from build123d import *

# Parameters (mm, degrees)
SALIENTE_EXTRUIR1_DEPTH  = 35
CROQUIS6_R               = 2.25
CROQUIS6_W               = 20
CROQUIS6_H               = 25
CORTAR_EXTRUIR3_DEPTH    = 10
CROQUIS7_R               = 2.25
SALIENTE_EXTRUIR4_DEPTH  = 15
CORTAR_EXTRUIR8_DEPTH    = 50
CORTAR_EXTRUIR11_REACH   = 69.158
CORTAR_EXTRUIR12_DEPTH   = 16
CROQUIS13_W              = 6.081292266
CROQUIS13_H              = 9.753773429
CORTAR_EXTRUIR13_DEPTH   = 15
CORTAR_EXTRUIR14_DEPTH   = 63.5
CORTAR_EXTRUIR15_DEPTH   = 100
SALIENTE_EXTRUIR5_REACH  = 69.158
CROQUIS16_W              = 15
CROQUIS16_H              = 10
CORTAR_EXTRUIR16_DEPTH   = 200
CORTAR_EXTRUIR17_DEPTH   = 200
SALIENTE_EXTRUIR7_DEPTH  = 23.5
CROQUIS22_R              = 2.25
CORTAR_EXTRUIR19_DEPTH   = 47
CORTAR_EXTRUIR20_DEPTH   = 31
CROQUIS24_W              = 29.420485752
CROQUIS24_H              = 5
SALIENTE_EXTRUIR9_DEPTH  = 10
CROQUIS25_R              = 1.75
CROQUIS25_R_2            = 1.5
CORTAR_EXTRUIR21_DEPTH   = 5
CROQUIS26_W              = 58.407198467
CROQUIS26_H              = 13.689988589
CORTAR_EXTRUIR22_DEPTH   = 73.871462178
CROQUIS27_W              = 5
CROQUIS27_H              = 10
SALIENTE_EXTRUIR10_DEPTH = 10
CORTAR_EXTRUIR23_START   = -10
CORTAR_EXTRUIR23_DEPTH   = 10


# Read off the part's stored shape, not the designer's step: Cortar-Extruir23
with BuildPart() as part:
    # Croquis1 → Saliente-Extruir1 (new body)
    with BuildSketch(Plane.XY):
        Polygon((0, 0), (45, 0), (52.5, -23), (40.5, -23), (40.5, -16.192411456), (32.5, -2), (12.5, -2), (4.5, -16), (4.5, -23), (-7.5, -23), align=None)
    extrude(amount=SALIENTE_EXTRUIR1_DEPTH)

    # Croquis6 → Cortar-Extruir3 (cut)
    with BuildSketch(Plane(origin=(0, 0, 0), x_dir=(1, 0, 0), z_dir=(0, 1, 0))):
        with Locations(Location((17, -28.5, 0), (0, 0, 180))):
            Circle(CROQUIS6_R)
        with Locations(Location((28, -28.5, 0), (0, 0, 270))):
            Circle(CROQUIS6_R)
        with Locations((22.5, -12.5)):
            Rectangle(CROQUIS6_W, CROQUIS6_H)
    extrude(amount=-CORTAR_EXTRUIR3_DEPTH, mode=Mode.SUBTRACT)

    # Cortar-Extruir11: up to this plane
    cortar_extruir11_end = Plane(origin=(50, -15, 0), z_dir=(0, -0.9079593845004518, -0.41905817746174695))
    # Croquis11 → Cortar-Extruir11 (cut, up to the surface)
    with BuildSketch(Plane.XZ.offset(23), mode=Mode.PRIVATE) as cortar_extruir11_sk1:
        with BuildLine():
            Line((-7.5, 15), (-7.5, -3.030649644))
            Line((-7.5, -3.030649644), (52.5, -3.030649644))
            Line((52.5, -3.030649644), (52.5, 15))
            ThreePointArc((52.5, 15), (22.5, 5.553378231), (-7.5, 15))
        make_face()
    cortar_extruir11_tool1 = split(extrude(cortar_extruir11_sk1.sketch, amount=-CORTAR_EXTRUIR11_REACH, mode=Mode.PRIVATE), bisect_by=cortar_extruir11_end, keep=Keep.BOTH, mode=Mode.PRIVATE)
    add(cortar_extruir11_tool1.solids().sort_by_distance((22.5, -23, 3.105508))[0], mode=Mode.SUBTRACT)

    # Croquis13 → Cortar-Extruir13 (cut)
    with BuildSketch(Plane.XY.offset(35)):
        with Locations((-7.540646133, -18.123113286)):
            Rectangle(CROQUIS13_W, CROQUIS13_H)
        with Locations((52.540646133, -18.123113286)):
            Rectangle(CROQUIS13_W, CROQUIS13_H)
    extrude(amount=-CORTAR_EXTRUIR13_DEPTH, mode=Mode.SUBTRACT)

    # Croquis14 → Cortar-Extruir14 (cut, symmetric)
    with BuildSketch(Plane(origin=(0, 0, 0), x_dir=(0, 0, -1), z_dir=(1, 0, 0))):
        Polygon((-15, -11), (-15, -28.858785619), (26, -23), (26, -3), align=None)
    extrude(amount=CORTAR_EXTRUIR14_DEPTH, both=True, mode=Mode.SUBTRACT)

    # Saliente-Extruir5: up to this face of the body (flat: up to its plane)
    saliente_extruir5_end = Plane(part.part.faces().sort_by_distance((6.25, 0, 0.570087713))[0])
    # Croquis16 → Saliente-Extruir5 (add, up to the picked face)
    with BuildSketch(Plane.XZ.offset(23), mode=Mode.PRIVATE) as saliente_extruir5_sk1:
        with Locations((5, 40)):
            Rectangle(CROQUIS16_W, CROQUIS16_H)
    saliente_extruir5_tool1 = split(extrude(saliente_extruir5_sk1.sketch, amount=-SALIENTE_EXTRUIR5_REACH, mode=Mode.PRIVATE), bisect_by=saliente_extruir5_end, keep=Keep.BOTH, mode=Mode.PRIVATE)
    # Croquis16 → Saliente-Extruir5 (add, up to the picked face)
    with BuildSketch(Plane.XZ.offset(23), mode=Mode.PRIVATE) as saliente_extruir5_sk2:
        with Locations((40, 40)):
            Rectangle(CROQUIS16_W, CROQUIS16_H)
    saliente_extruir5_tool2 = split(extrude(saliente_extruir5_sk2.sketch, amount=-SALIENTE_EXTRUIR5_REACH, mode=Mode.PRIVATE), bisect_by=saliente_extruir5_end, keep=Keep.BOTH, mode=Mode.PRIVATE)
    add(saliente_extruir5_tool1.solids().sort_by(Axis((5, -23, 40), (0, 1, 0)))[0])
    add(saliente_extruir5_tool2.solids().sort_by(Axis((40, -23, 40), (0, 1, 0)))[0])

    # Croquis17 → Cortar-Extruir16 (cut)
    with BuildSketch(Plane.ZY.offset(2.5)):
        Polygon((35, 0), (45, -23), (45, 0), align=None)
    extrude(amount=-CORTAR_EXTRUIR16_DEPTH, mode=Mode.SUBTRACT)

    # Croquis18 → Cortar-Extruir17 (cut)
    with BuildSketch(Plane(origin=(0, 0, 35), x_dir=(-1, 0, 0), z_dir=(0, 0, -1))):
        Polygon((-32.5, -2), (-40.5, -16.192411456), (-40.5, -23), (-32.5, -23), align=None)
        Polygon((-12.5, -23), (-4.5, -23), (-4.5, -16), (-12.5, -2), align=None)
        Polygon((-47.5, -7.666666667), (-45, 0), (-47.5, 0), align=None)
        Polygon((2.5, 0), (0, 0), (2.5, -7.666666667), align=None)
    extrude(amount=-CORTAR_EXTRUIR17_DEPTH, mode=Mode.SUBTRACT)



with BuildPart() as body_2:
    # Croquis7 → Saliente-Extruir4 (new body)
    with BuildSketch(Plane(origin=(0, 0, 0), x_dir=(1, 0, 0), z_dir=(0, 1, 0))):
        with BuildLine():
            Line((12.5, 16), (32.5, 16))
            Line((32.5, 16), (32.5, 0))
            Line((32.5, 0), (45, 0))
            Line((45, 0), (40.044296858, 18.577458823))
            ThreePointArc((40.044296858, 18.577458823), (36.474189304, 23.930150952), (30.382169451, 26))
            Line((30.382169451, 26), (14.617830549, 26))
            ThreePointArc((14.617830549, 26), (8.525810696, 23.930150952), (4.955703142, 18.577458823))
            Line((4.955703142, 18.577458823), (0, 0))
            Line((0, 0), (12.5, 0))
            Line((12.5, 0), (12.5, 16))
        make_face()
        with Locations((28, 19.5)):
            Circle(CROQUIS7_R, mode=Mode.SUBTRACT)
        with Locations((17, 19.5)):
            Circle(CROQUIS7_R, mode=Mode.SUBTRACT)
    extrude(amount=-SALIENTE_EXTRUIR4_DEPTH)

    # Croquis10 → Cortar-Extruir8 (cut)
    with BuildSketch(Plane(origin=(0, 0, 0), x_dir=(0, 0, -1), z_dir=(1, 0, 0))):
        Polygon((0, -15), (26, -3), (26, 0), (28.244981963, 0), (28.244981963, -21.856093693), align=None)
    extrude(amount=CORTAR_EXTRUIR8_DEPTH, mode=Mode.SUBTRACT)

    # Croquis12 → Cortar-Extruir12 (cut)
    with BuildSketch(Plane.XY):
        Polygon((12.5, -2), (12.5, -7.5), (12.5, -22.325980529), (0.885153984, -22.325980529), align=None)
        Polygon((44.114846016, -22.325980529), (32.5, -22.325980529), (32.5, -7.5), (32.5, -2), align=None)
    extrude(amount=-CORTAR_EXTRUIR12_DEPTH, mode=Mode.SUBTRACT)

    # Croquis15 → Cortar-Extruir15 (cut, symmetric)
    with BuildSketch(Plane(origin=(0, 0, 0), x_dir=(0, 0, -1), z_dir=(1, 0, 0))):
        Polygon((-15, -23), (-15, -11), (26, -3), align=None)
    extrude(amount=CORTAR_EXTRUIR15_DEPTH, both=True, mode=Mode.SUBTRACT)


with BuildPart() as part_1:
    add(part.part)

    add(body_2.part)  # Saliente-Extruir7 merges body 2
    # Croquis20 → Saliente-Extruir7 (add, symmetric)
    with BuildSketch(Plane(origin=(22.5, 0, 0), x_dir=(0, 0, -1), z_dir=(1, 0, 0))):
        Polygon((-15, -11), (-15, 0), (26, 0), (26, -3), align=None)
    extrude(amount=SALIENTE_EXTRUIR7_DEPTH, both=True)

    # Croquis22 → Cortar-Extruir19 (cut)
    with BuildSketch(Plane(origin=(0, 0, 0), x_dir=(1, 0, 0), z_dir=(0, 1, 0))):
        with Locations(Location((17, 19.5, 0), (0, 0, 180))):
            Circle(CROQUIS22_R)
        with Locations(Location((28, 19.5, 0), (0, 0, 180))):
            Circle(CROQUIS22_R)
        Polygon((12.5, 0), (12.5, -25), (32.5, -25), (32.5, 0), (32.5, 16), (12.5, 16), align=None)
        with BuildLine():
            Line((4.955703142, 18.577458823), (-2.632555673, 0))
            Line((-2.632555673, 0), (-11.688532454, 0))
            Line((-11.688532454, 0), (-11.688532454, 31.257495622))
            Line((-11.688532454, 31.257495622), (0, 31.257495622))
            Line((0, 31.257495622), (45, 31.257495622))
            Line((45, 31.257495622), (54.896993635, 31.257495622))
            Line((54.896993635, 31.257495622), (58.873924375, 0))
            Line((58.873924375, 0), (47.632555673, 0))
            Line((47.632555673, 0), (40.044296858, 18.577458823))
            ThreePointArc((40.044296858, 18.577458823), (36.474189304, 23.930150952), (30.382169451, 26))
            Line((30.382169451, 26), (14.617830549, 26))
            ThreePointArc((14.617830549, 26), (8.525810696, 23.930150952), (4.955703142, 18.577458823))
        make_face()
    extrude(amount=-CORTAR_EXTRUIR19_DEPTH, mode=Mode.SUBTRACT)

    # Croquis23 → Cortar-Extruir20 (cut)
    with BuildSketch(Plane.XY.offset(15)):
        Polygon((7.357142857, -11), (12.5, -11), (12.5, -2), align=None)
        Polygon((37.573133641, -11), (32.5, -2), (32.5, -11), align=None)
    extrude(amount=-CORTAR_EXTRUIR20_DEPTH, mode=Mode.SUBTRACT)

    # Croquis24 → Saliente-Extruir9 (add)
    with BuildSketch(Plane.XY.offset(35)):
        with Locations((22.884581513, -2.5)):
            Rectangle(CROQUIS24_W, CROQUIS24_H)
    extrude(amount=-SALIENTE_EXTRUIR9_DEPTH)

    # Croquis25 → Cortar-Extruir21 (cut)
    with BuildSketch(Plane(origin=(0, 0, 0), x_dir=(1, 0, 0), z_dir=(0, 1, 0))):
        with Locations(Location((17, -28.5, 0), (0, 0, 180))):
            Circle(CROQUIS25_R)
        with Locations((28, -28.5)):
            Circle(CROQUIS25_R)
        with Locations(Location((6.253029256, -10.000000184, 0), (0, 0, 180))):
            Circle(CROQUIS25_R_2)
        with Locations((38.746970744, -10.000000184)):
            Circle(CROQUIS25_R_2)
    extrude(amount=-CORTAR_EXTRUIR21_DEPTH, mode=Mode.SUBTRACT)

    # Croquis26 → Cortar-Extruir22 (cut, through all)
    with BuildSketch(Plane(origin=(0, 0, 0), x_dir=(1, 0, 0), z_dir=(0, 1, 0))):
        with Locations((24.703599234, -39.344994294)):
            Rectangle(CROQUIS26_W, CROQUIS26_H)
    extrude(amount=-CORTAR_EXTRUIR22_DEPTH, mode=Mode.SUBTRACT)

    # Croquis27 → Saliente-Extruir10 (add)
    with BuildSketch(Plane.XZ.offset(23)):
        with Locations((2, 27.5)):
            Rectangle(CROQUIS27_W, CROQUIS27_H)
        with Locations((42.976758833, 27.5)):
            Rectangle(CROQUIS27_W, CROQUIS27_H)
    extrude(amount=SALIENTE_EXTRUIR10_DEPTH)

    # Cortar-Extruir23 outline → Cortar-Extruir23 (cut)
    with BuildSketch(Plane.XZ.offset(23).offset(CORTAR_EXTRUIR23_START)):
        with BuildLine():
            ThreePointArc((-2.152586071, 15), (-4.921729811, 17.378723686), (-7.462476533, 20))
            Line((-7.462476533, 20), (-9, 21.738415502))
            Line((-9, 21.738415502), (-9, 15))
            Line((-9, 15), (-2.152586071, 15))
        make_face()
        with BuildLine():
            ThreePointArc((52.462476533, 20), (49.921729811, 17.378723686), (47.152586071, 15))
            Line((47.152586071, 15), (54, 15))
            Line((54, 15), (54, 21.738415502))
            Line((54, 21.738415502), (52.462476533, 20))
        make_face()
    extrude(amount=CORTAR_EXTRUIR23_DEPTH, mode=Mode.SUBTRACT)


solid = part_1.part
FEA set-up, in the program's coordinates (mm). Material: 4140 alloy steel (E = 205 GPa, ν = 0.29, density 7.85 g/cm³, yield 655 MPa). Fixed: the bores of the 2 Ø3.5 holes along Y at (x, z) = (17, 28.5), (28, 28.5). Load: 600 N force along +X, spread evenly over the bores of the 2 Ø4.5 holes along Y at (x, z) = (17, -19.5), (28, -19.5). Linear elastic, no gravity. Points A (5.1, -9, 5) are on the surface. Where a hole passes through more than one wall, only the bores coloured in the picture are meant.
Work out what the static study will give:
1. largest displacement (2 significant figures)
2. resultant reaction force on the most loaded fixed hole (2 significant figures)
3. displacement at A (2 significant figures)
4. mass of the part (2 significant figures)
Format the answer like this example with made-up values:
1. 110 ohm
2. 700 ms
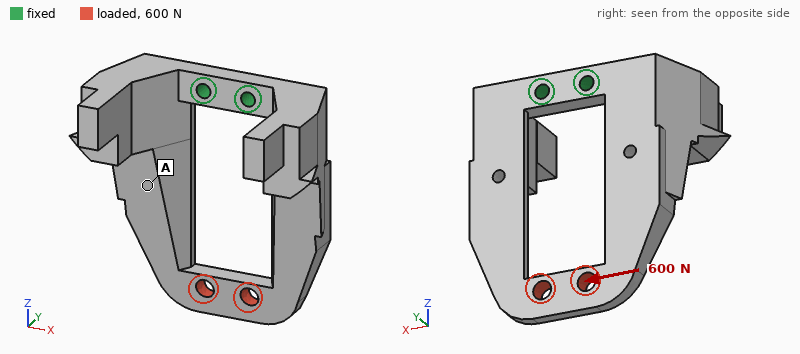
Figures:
1. 0.14 mm
2. 960 N
3. 0.070 mm
4. 140 g
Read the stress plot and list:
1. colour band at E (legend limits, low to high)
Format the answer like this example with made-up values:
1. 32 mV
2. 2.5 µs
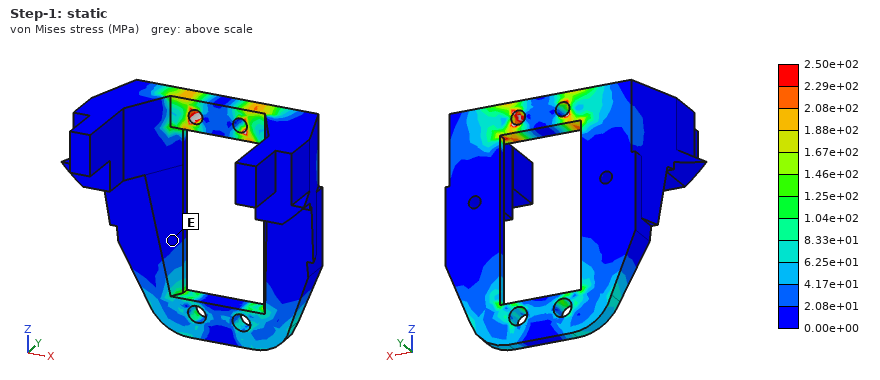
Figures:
1. 0.00e+00 to 2.08e+01 MPa
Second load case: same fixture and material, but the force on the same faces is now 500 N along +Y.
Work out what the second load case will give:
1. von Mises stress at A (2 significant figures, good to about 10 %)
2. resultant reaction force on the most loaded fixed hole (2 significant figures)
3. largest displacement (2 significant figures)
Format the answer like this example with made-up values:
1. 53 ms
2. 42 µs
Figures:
1. 44 MPa
2. 260 N
3. 0.34 mm
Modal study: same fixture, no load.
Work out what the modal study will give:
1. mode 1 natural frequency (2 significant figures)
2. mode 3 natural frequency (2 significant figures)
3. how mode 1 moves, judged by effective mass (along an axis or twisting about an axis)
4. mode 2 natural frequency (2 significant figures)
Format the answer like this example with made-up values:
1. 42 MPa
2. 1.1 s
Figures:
1. 1200 Hz
2. 1800 Hz
3. along Y
4. 1800 Hz
